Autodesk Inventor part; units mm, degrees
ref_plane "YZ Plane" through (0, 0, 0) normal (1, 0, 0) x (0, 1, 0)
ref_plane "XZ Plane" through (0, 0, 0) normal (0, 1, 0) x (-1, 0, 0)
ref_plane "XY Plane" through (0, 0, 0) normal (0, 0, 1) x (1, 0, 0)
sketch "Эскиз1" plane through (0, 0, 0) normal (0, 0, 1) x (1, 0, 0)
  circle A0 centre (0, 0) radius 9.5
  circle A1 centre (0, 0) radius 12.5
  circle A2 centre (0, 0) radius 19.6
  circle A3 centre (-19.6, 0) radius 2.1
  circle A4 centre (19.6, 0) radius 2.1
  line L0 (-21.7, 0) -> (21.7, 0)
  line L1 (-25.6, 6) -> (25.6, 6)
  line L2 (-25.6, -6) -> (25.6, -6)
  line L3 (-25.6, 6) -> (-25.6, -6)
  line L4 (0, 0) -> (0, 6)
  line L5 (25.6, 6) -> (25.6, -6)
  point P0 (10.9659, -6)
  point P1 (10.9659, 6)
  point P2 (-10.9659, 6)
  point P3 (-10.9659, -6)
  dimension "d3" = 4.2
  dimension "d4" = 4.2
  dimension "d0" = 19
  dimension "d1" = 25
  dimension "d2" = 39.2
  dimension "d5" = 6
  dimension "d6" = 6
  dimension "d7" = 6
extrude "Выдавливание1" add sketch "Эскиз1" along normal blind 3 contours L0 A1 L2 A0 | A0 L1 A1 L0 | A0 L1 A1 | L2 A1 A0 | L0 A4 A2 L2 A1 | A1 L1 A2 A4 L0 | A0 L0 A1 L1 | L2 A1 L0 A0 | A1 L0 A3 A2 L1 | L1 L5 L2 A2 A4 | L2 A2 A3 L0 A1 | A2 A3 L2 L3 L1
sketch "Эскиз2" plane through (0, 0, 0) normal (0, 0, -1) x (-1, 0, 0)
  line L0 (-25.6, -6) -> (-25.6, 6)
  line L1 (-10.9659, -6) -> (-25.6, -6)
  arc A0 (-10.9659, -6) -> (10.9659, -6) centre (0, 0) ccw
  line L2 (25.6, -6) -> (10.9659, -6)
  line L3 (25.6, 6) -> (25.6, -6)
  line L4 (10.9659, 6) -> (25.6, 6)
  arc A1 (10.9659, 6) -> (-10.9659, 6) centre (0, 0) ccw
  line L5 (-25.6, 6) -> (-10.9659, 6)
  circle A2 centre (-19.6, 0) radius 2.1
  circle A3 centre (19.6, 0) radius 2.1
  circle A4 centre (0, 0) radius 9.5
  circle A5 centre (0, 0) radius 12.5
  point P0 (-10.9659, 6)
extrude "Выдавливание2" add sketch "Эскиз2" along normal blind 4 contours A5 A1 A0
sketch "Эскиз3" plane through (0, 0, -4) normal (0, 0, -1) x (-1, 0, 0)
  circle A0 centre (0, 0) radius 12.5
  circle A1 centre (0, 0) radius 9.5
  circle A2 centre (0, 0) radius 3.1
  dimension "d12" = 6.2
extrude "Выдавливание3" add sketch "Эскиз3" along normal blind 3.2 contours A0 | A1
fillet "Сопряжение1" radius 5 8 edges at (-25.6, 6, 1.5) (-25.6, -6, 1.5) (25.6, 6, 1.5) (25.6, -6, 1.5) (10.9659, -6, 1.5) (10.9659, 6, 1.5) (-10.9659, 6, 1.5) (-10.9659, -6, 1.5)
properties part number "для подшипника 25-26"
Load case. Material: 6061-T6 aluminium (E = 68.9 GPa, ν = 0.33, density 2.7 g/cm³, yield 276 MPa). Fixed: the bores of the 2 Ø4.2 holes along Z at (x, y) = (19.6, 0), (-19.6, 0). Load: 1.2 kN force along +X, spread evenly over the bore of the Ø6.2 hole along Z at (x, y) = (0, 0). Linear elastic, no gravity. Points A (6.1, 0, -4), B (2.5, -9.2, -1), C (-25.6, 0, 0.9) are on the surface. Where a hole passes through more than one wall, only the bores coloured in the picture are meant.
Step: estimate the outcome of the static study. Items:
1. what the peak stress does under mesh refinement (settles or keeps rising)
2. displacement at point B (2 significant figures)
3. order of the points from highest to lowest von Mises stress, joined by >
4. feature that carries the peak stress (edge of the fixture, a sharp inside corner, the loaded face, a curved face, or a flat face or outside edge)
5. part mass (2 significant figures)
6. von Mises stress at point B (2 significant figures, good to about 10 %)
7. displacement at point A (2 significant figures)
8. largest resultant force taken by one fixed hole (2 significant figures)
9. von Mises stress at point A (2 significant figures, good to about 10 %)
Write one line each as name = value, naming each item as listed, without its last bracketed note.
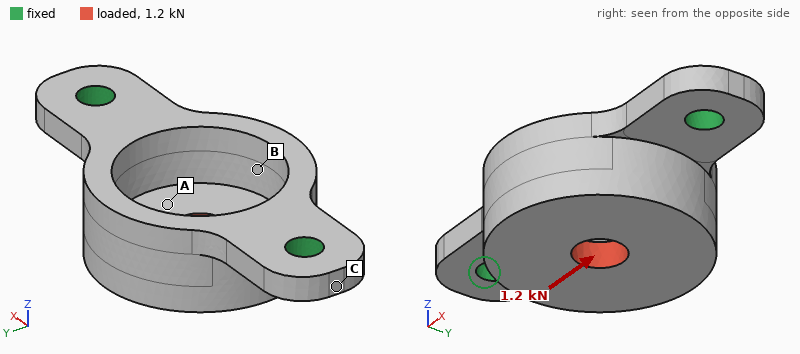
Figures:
what the peak stress does under mesh refinement = keeps rising
displacement at point B = 6.4 µm
order of the points from highest to lowest von Mises stress, joined by > = A > B > C
feature that carries the peak stress = edge of the fixture
part mass = 10 g
von Mises stress at point B = 13 MPa
displacement at point A = 10.0 µm
largest resultant force taken by one fixed hole = 660 N
von Mises stress at point A = 25 MPa
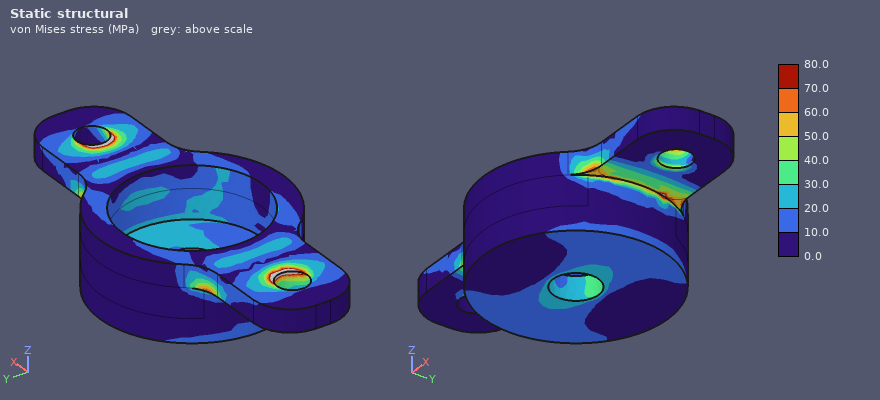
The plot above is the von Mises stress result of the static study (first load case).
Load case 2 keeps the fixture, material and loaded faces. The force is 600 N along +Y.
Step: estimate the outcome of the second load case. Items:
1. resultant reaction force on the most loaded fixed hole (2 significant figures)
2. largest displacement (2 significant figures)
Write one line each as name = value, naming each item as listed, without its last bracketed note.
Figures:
resultant reaction force on the most loaded fixed hole = 300 N
largest displacement = 84 µm
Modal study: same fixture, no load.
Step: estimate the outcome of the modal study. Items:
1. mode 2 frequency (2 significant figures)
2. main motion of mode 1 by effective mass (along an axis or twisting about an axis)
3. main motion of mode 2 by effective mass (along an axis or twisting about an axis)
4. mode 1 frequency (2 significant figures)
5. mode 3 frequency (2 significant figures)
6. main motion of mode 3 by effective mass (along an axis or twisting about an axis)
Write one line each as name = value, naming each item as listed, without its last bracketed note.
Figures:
mode 2 frequency = 12 kHz
main motion of mode 1 by effective mass = along Y
main motion of mode 2 by effective mass = along Z
mode 1 frequency = 5600 Hz
mode 3 frequency = 21 kHz
main motion of mode 3 by effective mass = along X
